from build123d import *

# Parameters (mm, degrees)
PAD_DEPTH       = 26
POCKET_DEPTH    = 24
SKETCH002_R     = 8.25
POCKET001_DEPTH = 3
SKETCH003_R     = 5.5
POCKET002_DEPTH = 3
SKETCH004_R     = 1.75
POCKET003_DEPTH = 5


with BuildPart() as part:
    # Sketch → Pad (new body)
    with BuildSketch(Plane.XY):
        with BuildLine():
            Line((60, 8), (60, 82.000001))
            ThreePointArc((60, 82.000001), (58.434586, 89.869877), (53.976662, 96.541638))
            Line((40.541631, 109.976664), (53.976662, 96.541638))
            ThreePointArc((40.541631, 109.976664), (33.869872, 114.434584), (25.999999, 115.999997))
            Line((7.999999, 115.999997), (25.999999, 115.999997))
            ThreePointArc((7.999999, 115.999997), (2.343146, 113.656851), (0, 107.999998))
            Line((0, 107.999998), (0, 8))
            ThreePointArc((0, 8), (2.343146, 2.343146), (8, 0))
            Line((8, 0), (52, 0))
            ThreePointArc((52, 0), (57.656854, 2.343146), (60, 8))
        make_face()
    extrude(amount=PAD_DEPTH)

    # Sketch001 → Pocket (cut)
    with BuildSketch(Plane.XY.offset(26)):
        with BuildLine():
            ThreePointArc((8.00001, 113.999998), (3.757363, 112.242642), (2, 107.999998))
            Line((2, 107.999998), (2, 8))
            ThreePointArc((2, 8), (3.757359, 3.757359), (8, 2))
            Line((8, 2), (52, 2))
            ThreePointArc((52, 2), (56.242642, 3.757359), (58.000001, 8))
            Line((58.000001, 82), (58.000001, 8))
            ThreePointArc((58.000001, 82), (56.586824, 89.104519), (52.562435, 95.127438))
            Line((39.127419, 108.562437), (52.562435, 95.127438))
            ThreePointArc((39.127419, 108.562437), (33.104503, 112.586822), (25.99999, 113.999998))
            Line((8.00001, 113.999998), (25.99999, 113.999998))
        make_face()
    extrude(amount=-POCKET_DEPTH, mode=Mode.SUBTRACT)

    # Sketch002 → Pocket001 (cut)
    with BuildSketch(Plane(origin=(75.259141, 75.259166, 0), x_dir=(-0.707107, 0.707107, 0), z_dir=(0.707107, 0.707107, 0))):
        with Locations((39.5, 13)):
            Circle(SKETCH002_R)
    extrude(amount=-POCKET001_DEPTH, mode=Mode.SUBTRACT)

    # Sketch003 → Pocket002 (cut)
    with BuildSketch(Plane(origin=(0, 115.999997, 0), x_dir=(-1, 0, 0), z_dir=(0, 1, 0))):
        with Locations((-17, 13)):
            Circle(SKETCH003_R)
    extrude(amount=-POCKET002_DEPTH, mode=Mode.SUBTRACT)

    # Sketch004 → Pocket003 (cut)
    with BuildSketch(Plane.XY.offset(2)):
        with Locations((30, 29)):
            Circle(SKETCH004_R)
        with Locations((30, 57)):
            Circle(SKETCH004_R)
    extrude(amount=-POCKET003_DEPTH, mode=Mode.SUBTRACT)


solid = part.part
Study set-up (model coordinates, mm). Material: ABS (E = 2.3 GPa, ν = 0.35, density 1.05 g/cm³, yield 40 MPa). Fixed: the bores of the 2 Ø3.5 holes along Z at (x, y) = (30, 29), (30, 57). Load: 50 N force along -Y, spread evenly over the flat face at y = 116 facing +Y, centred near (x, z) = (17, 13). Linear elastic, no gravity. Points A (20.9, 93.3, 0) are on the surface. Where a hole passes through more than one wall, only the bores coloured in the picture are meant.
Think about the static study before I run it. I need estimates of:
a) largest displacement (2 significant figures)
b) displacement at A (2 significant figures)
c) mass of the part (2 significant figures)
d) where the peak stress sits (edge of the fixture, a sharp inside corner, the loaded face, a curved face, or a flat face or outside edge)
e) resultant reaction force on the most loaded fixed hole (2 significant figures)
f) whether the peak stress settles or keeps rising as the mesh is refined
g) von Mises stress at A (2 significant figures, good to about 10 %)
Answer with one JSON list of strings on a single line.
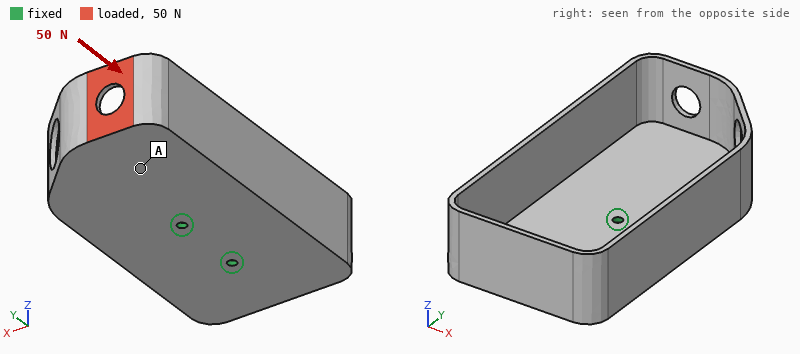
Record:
["1.5 mm", "0.64 mm", "29 g", "edge of the fixture", "39 N", "keeps rising", "1.1 MPa"]
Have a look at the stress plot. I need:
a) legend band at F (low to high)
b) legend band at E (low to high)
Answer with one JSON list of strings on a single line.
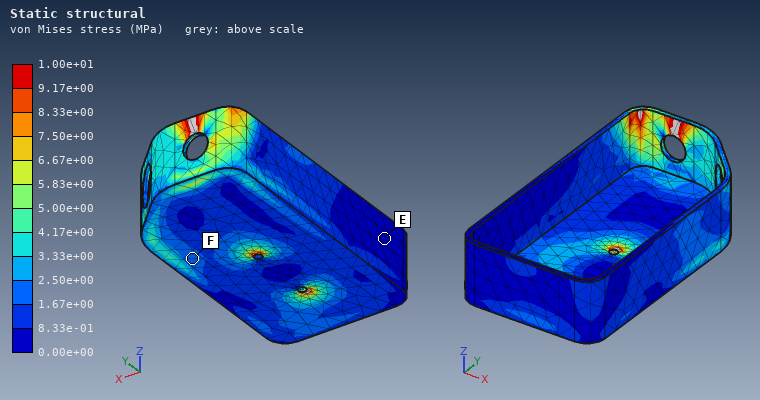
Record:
["1.67e+00 to 2.50e+00 MPa", "0.00e+00 to 8.33e-01 MPa"]
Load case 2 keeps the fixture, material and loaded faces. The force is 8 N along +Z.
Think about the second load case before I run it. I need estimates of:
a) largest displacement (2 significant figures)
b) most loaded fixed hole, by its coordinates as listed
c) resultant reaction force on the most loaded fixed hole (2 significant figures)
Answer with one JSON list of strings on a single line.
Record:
["1.5 mm", "(30, 57)", "19 N"]
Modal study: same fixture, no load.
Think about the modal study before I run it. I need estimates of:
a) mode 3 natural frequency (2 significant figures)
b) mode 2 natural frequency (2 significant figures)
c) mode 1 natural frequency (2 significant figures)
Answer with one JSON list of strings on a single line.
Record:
["260 Hz", "170 Hz", "150 Hz"]
